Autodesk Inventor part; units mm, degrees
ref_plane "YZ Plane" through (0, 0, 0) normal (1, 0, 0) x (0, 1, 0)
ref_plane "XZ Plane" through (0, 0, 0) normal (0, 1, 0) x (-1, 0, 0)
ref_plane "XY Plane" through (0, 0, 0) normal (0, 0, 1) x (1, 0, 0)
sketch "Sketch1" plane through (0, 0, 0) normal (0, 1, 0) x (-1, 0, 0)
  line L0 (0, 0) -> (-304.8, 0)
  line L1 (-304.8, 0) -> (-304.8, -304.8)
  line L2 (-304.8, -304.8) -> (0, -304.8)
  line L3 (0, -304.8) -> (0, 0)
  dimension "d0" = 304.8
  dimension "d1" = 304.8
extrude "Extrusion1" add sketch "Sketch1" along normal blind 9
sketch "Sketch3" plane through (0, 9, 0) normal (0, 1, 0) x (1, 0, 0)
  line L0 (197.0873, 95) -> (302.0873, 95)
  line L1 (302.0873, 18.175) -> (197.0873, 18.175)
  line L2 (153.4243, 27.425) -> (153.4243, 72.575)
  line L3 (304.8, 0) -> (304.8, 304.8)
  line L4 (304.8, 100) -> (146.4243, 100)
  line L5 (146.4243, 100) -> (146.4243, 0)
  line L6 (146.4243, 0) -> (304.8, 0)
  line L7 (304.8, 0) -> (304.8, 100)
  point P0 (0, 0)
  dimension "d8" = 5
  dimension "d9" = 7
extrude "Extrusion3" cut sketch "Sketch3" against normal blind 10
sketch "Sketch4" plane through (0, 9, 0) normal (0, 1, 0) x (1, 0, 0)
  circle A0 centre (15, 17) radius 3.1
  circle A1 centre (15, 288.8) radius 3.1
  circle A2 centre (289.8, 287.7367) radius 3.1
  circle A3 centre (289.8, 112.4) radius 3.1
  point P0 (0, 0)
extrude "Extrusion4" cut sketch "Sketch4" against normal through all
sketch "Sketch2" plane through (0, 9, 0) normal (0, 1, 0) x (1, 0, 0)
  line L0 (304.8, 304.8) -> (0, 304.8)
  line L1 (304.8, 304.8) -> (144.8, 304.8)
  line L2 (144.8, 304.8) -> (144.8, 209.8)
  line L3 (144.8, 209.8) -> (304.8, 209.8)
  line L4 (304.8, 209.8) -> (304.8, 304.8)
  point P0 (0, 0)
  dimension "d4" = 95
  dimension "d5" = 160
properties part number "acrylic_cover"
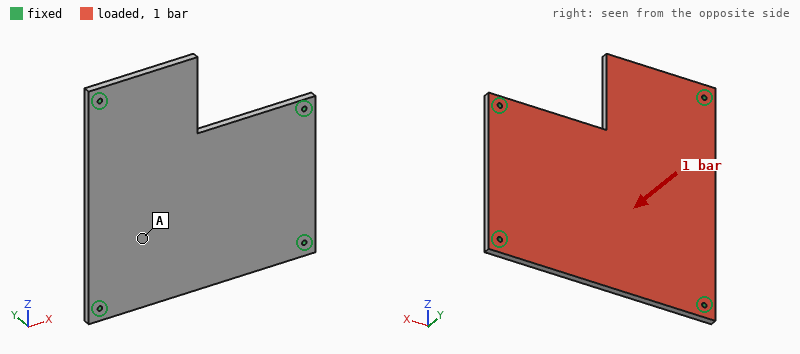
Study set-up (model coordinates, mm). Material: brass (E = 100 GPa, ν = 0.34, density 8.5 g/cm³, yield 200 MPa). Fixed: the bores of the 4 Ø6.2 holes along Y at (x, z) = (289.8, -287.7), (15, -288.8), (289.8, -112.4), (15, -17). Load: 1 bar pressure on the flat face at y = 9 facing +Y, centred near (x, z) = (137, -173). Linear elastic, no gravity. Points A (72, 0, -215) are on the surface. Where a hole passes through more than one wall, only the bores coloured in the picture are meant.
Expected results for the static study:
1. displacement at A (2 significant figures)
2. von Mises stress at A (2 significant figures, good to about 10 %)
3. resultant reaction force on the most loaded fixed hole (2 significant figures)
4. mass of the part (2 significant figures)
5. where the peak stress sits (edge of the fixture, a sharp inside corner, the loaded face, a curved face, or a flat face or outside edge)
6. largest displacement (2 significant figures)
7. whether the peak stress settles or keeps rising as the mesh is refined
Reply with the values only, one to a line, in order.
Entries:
0.46 mm
22 MPa
2.2 kN
5.9 kg
edge of the fixture
0.69 mm
keeps rising
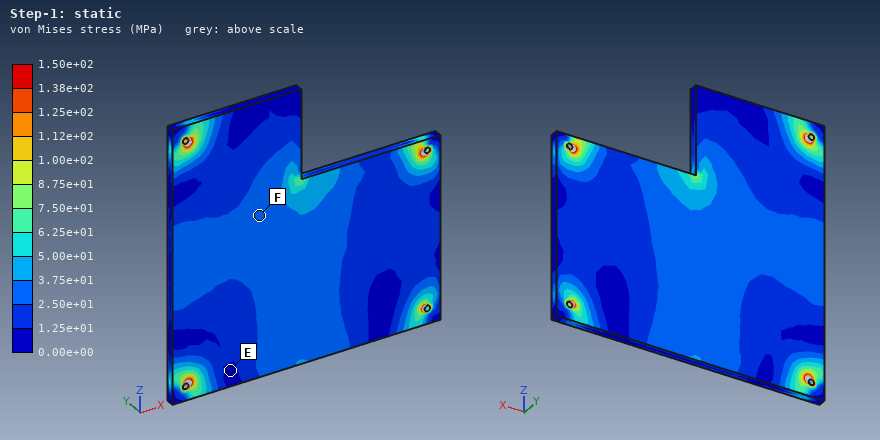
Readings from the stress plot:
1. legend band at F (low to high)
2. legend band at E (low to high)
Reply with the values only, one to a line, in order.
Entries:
2.50e+01 to 3.75e+01 MPa
0.00e+00 to 1.25e+01 MPa
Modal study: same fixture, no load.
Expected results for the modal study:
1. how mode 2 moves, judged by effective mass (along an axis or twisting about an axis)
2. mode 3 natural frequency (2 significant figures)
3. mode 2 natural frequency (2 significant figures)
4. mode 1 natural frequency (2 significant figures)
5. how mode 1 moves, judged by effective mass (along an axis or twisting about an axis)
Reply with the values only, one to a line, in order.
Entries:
twisting about X
460 Hz
420 Hz
260 Hz
along Y
